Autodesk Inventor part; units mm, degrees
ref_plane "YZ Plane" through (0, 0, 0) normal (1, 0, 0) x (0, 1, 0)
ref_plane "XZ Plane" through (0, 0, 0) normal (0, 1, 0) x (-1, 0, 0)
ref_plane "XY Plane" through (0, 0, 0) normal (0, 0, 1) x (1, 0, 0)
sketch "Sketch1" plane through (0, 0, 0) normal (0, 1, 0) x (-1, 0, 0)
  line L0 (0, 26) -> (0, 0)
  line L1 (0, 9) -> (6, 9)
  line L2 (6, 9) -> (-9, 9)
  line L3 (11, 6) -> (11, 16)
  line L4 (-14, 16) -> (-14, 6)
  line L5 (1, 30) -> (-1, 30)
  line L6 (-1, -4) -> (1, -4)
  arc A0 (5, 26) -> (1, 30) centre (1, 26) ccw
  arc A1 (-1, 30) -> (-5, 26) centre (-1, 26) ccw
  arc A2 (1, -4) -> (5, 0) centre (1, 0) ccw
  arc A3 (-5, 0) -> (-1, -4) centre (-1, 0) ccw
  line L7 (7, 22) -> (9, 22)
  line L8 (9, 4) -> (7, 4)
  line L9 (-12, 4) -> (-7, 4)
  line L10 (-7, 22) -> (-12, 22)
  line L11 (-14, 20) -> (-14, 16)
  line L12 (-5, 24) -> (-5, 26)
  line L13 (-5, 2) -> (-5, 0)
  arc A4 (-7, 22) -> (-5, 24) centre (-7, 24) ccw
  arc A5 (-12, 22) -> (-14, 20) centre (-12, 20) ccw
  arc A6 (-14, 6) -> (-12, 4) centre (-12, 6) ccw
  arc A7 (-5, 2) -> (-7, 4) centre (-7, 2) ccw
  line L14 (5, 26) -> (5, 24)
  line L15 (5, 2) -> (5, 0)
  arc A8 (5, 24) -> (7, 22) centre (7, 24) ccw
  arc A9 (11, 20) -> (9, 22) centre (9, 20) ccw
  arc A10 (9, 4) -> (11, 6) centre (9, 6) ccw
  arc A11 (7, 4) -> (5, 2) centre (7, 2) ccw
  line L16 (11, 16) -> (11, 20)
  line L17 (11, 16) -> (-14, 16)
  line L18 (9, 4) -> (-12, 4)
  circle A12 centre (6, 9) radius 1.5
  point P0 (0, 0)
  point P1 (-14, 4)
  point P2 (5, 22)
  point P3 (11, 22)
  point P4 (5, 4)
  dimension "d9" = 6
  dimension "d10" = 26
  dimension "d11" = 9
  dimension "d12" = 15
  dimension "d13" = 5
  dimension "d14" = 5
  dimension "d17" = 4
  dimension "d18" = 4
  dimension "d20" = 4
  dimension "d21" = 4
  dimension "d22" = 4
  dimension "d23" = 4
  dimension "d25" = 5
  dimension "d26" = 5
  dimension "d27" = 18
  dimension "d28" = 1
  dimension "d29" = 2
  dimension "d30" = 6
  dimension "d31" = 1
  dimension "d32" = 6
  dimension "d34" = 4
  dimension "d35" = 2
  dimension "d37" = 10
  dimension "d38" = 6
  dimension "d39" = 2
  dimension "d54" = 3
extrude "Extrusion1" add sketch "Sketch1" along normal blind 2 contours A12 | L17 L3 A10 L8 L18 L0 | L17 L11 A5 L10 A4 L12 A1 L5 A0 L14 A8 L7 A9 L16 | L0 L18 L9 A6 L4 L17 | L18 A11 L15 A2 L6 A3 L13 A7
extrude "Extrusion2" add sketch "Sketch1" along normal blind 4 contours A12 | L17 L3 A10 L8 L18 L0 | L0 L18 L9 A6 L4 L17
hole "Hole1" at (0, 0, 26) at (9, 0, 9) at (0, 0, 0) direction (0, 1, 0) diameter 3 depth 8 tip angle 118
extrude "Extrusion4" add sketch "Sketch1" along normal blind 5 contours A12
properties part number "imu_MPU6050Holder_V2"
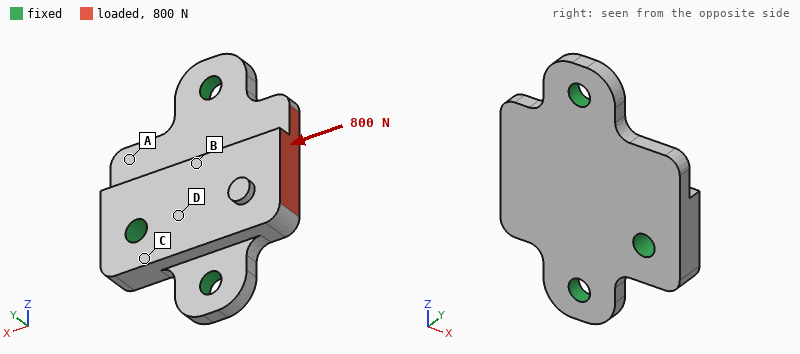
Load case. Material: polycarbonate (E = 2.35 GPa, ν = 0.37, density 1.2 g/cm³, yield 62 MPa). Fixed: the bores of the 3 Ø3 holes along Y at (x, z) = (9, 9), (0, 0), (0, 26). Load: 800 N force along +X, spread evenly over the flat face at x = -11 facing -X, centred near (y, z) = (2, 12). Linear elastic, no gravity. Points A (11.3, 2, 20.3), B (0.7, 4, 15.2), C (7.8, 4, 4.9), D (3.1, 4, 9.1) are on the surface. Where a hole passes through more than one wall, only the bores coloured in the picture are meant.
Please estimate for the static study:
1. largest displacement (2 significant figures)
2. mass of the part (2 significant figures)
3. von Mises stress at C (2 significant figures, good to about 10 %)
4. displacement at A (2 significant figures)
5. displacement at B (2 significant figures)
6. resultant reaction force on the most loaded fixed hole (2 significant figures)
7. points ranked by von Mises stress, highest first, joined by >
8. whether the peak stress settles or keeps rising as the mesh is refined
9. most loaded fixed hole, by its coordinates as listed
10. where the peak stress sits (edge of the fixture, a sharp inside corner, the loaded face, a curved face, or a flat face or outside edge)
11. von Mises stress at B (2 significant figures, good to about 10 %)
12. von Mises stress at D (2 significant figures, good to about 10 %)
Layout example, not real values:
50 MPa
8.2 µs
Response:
0.18 mm
2.1 g
6.6 MPa
0.050 mm
0.072 mm
530 N
D > B > C > A
keeps rising
(9, 9)
edge of the fixture
13 MPa
18 MPa
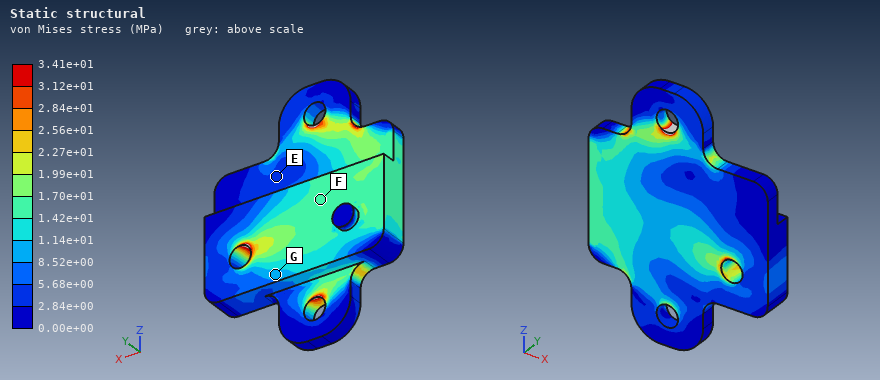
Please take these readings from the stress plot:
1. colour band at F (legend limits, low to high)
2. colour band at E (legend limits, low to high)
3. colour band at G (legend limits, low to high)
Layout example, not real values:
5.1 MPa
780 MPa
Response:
1.42e+01 to 1.70e+01 MPa
2.84e+00 to 5.68e+00 MPa
8.52e+00 to 1.14e+01 MPa
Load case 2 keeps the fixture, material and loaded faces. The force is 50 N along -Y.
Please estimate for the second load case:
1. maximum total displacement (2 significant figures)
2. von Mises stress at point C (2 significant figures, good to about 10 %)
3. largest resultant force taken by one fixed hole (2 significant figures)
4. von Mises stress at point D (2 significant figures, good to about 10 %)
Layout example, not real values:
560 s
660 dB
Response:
0.41 mm
5.2 MPa
59 N
11 MPa
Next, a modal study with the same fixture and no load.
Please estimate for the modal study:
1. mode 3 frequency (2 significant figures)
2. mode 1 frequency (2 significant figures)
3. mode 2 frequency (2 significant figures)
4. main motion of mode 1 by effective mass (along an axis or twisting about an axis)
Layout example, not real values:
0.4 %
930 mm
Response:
8700 Hz
3400 Hz
8300 Hz
along Y
